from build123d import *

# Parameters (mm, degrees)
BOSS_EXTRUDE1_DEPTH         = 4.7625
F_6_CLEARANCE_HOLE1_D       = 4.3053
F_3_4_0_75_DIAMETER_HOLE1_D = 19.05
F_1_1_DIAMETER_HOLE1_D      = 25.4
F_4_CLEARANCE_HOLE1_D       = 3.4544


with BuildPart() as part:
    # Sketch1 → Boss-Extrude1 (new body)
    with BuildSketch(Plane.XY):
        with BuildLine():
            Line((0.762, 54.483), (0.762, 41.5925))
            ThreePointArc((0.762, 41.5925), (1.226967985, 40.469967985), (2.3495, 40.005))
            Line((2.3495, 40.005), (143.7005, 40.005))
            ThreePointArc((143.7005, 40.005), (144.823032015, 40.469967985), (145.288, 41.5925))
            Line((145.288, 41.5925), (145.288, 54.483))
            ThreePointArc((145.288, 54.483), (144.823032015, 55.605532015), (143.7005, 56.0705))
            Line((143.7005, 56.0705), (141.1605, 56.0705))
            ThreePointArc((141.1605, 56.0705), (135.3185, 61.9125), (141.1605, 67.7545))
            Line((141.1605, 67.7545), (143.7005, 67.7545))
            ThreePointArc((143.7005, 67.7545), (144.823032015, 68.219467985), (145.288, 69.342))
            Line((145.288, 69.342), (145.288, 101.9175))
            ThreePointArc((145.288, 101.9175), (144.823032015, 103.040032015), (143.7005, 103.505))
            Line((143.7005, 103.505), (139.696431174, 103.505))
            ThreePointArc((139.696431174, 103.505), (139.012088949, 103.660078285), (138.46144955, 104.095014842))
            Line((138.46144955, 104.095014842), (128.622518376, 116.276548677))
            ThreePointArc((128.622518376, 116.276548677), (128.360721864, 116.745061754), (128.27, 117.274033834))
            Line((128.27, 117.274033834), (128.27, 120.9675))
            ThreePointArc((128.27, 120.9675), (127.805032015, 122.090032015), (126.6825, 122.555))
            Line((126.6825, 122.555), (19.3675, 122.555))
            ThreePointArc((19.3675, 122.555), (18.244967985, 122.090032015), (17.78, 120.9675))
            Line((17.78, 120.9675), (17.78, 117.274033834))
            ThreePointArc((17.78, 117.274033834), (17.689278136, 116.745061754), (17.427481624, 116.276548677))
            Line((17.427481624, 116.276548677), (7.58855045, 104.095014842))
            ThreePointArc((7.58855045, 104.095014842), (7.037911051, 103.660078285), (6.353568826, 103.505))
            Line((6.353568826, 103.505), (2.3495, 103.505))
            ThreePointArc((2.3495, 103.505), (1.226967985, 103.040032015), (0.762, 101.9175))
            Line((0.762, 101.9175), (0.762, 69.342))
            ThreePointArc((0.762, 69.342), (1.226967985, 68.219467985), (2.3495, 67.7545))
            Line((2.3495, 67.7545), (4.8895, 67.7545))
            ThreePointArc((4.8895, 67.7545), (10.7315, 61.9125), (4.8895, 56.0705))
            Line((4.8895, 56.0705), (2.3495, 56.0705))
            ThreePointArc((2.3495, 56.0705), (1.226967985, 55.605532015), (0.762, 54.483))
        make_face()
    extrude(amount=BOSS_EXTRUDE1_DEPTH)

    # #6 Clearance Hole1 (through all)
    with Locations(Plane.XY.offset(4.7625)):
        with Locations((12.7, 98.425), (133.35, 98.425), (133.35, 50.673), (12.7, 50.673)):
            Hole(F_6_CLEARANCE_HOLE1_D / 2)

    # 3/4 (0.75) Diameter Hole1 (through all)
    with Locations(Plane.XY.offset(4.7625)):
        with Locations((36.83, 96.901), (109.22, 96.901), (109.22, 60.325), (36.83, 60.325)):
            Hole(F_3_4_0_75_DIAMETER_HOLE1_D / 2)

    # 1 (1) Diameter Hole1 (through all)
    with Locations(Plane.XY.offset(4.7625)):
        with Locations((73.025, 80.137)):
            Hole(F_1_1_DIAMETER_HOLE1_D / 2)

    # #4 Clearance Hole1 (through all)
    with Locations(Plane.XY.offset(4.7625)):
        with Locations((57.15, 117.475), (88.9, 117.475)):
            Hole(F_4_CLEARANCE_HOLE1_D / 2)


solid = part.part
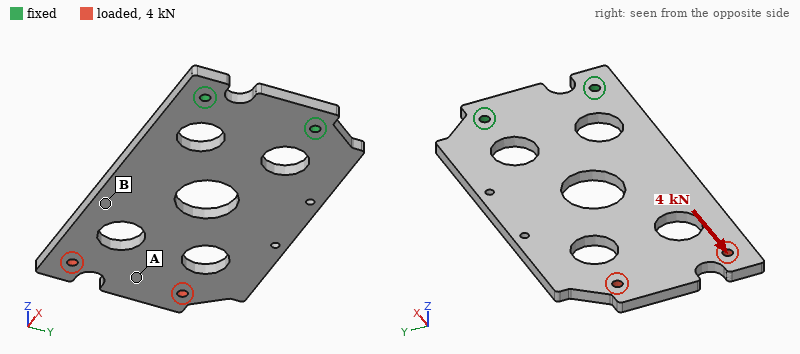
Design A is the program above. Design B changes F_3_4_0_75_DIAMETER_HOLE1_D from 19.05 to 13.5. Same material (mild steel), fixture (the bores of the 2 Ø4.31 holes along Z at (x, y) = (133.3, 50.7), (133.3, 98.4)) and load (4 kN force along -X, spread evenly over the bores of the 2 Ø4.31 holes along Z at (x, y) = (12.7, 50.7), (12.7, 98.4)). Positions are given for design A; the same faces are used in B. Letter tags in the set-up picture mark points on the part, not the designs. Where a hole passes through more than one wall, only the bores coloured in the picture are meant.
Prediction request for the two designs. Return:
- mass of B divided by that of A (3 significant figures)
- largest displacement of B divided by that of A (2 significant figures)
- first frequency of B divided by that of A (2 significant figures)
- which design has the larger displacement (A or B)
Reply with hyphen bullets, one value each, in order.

- 1.06
- 0.88
- 1.0
- A
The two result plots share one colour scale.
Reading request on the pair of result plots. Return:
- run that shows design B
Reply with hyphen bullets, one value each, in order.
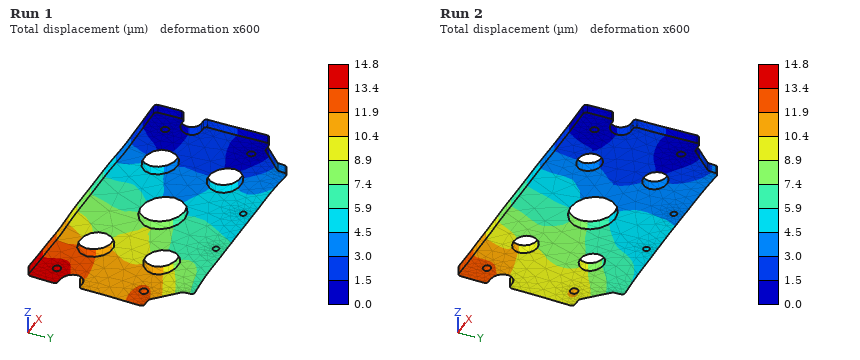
- Run 2
